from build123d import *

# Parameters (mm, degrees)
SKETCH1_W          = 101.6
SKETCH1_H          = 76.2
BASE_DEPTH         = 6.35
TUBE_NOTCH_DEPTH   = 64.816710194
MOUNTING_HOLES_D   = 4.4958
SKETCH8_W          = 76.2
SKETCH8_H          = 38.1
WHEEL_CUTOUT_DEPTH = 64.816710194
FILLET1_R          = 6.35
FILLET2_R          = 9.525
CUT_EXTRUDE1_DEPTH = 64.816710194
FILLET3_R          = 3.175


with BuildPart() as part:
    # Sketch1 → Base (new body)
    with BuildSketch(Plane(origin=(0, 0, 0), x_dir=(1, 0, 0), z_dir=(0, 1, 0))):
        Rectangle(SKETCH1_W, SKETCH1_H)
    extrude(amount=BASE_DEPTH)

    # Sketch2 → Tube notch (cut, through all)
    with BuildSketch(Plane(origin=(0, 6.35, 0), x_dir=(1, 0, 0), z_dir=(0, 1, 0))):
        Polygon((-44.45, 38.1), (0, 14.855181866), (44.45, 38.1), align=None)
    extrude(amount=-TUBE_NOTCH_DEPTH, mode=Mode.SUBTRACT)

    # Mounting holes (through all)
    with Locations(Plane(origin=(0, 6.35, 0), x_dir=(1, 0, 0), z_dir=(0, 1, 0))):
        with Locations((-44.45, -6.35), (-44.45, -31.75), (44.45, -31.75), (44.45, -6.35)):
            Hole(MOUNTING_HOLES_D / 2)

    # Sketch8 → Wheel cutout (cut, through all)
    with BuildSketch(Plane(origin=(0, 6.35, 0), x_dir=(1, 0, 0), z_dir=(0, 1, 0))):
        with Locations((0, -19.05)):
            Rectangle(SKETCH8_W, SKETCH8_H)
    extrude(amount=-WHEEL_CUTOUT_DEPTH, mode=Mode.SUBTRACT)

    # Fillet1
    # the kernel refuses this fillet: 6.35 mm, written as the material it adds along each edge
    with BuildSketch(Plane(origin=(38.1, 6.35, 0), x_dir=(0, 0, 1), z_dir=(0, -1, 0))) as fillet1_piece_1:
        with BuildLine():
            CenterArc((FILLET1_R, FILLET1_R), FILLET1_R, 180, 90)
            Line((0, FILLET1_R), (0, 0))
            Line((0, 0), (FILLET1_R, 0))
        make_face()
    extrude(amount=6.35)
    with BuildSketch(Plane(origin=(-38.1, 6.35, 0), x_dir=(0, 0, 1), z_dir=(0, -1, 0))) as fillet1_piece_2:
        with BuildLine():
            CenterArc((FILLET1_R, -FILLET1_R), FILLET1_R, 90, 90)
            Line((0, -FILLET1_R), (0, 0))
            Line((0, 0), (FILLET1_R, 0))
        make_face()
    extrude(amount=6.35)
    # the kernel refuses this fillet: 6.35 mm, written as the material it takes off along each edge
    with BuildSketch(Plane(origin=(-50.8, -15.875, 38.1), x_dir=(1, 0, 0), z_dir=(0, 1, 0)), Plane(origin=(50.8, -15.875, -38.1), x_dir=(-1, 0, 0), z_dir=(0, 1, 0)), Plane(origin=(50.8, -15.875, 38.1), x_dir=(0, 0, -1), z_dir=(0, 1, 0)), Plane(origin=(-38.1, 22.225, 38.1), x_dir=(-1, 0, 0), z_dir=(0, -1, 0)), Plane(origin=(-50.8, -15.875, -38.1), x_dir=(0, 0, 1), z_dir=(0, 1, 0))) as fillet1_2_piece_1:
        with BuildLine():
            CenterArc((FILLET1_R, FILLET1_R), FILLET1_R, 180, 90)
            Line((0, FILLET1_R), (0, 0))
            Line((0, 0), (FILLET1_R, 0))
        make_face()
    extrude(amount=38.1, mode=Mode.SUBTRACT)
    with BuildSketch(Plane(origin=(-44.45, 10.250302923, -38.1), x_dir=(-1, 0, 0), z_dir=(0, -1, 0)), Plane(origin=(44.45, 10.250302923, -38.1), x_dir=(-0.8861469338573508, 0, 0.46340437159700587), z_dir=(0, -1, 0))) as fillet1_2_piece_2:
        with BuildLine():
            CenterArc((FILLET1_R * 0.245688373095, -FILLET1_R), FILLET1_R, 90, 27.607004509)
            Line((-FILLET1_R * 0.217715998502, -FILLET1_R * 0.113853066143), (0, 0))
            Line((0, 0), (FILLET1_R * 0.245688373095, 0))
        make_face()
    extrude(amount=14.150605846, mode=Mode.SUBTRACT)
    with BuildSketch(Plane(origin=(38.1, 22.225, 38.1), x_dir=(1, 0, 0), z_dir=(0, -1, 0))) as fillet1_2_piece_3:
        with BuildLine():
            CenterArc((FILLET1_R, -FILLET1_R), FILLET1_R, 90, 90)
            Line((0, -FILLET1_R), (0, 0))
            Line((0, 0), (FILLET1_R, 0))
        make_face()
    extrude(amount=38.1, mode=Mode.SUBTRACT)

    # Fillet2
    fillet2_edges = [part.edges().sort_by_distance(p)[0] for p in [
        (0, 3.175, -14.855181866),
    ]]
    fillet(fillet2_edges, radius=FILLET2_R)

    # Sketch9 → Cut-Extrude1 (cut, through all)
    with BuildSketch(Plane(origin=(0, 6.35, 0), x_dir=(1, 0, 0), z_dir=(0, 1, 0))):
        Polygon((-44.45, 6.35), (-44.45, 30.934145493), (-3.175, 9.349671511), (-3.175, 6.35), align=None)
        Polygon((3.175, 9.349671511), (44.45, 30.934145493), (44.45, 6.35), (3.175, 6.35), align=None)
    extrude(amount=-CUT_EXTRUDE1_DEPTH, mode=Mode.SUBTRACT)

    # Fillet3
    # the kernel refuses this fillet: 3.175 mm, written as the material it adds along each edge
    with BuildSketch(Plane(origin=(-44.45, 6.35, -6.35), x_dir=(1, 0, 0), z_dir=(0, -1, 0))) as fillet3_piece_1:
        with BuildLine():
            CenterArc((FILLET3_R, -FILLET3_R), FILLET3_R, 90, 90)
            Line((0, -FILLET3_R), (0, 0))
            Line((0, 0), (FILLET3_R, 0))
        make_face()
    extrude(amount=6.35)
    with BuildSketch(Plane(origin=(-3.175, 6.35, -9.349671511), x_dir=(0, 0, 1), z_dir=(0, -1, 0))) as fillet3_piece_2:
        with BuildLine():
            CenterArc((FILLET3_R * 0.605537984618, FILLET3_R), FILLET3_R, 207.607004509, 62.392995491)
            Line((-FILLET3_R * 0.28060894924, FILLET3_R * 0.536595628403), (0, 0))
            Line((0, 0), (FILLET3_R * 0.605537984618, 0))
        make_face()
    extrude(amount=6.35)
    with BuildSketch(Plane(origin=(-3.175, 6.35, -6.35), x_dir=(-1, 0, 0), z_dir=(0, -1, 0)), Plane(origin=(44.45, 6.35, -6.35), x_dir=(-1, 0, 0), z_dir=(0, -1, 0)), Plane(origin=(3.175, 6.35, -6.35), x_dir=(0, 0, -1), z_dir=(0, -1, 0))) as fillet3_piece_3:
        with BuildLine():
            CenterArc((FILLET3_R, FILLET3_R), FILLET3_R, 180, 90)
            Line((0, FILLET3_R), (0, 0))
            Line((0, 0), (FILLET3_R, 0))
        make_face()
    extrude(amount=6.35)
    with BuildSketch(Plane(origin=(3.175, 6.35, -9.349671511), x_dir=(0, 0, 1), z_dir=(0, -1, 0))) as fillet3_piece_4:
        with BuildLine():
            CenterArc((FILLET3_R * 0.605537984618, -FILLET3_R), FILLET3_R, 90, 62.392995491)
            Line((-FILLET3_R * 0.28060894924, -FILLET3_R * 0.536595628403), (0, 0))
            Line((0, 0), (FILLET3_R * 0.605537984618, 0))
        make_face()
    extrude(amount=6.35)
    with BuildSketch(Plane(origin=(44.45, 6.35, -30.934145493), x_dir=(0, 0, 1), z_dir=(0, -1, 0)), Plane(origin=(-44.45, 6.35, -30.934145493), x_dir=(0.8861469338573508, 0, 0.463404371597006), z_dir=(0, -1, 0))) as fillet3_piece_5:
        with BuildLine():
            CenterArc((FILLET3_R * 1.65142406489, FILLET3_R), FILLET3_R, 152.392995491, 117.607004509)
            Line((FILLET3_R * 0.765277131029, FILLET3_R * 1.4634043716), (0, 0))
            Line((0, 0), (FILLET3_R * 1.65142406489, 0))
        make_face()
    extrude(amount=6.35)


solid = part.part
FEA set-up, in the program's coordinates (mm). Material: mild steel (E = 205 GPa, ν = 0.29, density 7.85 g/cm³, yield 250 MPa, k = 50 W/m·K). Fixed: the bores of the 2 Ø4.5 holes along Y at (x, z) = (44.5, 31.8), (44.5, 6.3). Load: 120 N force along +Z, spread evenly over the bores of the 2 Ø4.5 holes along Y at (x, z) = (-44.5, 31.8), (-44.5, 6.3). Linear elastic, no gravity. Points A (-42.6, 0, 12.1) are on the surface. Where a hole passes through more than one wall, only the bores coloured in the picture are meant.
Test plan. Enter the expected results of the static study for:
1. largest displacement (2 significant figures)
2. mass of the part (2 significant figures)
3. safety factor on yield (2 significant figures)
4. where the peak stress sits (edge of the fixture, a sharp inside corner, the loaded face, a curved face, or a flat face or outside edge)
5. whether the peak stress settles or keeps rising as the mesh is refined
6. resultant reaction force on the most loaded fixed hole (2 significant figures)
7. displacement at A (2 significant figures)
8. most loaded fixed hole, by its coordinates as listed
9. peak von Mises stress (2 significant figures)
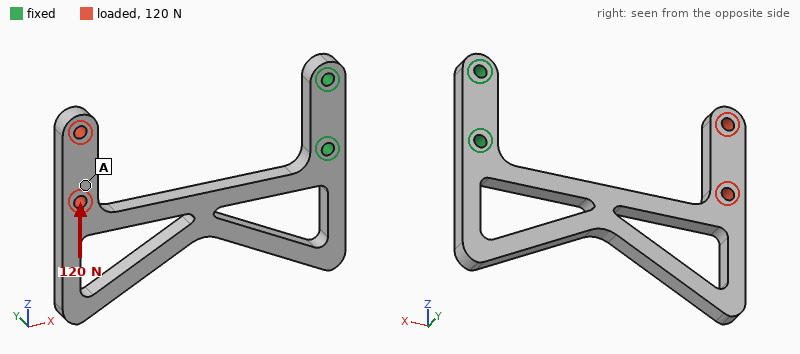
0.30 mm
130 g
1.7
a curved face
settles
200 N
0.24 mm
(44.5, 6.3)
150 MPa
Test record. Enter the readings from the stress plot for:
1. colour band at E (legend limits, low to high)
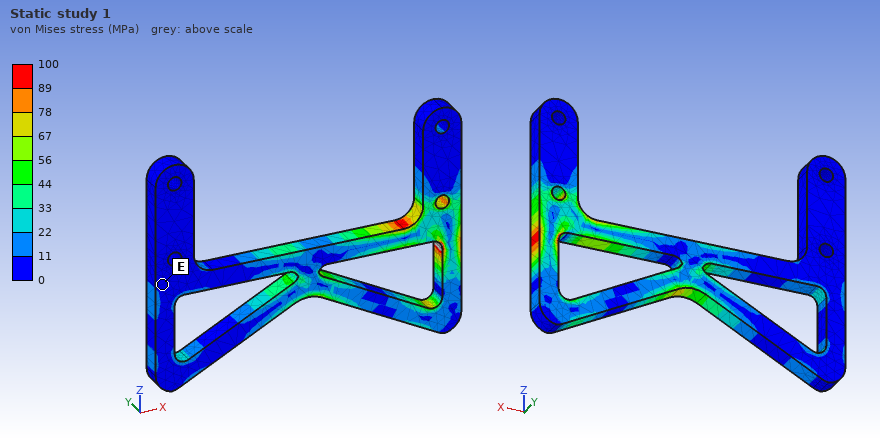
0 to 11 MPa
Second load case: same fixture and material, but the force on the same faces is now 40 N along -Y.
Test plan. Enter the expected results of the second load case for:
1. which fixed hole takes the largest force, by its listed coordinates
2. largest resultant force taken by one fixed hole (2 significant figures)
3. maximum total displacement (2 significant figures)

(44.5, 6.3)
41 N
0.32 mm
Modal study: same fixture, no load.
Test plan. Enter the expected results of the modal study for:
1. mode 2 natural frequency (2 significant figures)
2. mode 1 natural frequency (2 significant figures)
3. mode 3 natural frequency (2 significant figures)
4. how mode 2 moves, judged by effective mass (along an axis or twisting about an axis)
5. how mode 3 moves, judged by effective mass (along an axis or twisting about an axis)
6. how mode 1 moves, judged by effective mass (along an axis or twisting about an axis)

470 Hz
300 Hz
730 Hz
along Z
twisting about X
along Y
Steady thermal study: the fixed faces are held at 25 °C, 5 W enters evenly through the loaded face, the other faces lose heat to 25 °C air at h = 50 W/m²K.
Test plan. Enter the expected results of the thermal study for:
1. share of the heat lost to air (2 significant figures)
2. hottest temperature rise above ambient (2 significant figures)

94 %
39 K
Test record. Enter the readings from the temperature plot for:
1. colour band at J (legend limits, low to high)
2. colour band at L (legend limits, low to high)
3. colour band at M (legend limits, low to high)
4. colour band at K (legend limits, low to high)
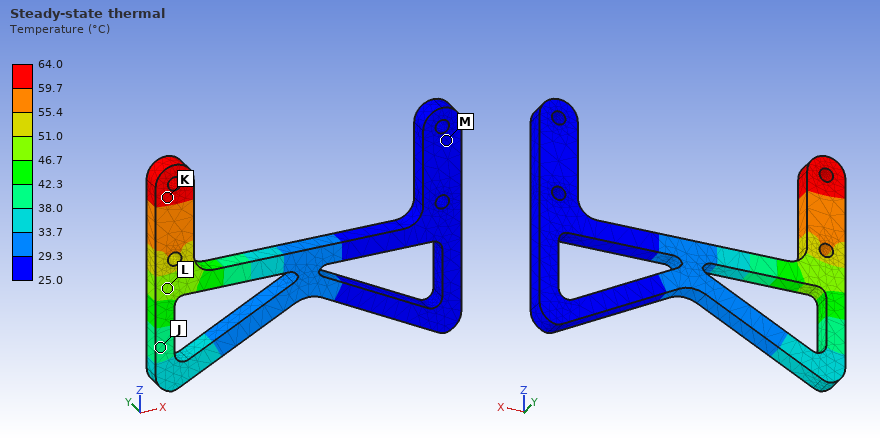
38.0 to 42.3 °C
46.7 to 51.0 °C
25.0 to 29.3 °C
59.7 to 64.0 °C
